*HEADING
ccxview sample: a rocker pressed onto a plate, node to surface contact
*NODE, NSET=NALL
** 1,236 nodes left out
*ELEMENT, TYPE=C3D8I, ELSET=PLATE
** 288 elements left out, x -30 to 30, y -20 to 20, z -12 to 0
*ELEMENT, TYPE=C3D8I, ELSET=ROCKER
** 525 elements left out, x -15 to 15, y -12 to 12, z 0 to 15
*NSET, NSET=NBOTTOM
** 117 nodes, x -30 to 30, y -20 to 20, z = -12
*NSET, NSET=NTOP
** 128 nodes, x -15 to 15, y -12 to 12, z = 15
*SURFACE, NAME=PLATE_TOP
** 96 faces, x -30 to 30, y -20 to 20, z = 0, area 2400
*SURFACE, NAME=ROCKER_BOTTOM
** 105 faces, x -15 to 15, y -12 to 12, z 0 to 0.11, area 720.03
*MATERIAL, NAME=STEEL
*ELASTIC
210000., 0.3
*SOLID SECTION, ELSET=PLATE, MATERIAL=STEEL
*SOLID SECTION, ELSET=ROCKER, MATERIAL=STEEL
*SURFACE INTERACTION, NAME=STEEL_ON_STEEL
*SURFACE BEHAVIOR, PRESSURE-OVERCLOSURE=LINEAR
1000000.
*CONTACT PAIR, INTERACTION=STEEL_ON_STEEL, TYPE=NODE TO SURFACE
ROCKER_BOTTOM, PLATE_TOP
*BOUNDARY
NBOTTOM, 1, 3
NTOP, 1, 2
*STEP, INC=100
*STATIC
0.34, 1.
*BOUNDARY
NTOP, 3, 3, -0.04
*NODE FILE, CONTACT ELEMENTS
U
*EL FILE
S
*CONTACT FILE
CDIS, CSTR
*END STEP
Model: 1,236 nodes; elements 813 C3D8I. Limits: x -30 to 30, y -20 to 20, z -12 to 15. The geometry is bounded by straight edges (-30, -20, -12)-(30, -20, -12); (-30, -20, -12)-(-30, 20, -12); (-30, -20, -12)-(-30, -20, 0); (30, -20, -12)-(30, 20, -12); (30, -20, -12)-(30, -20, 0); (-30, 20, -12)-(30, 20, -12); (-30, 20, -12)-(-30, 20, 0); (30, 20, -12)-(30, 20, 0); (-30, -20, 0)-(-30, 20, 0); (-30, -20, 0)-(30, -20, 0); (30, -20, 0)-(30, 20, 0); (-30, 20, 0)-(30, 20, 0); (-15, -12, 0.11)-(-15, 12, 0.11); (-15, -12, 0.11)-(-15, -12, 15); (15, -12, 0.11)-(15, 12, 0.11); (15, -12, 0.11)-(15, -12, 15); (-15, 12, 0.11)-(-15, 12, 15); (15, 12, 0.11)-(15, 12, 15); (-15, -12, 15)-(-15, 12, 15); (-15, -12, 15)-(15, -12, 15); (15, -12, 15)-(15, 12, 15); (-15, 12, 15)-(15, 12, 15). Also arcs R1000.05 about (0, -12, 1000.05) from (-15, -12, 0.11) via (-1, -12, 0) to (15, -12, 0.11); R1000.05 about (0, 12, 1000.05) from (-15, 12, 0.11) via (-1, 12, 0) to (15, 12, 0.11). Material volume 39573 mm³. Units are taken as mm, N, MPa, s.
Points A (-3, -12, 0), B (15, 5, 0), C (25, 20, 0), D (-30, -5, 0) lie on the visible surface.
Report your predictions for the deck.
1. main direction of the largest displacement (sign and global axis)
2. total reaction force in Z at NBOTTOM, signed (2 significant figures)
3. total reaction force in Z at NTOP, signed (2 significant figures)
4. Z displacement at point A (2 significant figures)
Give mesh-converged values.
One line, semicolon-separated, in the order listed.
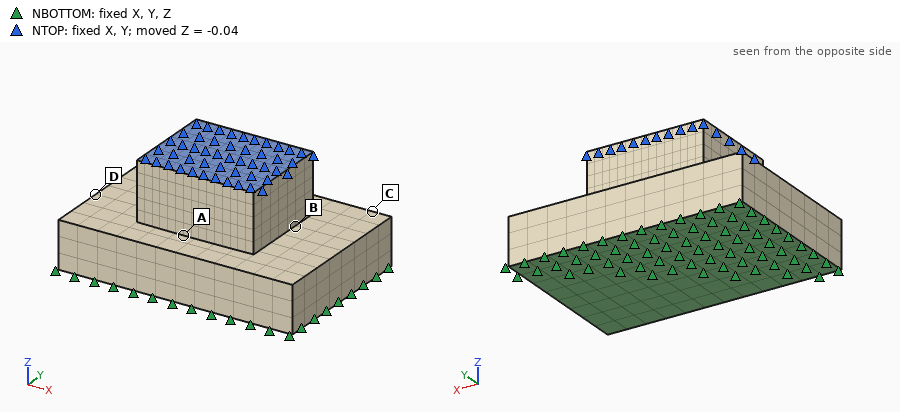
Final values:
-Z; 1.2e+05 N; -1.2e+05 N; -0.014 mm
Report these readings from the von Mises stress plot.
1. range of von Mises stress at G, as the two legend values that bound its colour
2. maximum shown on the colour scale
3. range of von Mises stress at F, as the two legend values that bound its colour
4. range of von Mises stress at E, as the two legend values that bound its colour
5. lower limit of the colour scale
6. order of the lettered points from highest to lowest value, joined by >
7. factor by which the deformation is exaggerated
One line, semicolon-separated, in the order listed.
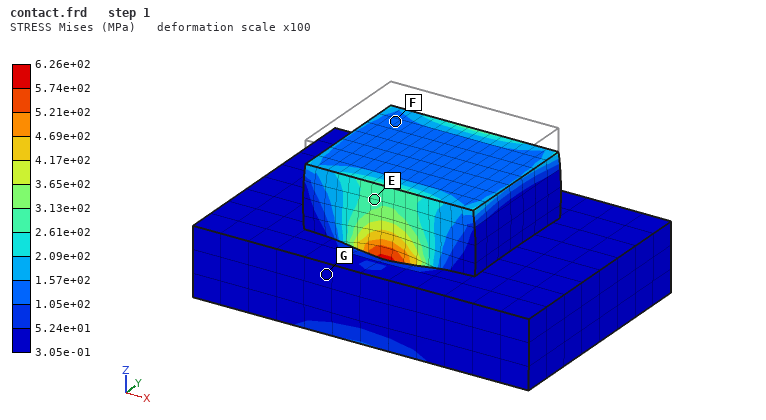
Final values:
3.05e-01 to 5.24e+01 MPa; 6.26e+02 MPa; 1.05e+02 to 1.57e+02 MPa; 2.61e+02 to 3.13e+02 MPa; 3.05e-01 MPa; E > F > G; 100
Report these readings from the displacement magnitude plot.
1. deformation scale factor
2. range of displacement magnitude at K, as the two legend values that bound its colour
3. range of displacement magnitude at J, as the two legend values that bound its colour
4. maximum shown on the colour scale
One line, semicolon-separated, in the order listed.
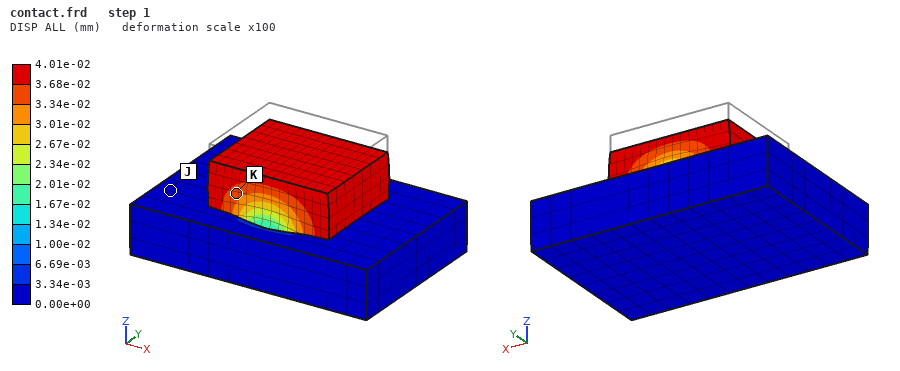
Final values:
100; 3.34e-02 to 3.68e-02 mm; 0.00e+00 to 3.34e-03 mm; 4.01e-02 mm
